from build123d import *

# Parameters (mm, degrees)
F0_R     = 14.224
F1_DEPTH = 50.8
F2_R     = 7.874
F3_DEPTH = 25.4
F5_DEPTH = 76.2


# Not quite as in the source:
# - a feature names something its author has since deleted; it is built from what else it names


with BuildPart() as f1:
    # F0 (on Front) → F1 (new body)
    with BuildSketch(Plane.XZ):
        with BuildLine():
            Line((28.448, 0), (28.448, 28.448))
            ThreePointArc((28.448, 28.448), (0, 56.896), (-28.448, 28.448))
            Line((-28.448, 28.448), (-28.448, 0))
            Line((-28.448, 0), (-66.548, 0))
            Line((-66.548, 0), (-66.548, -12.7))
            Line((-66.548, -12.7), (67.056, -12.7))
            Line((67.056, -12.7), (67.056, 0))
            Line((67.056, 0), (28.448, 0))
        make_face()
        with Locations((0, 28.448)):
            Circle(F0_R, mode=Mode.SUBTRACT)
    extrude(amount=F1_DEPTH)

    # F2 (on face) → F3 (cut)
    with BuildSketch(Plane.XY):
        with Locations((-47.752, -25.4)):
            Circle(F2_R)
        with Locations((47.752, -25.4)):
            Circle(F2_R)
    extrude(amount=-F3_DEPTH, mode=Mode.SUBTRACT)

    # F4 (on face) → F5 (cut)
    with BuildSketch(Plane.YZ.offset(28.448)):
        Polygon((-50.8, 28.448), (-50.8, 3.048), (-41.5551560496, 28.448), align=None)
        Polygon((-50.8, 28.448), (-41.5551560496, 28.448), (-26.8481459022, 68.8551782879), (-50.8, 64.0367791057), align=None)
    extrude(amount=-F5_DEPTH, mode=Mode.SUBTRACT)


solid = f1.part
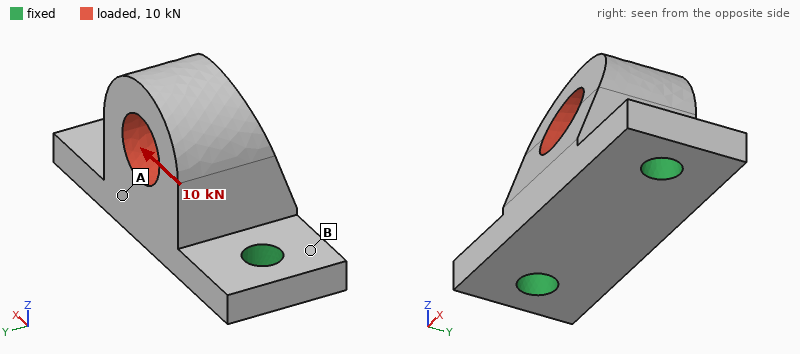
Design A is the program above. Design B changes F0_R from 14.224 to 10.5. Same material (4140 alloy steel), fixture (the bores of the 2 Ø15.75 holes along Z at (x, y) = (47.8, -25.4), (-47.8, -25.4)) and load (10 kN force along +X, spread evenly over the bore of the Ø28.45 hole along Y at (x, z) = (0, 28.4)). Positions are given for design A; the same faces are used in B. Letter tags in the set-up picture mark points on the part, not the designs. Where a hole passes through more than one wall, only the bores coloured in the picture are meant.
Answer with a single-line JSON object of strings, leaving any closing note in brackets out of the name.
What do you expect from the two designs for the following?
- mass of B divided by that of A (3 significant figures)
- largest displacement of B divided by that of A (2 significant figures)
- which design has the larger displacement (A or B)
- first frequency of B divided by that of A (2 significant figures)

{"mass of B divided by that of A": "1.07", "largest displacement of B divided by that of A": "0.88", "which design has the larger displacement": "A", "first frequency of B divided by that of A": "0.94"}
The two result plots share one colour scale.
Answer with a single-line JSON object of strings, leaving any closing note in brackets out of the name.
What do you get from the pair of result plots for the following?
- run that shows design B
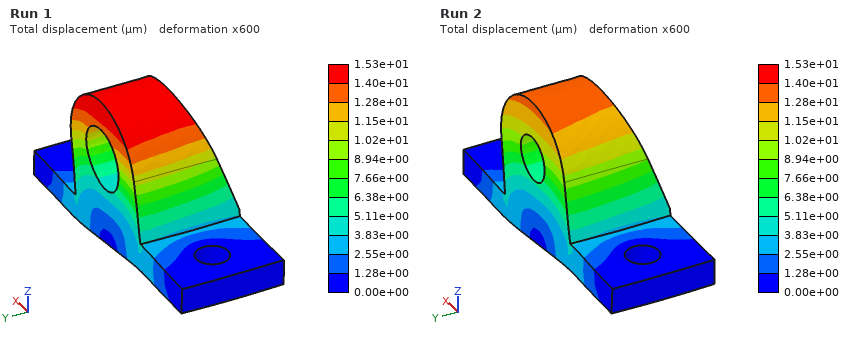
{"run that shows design B": "Run 2"}
